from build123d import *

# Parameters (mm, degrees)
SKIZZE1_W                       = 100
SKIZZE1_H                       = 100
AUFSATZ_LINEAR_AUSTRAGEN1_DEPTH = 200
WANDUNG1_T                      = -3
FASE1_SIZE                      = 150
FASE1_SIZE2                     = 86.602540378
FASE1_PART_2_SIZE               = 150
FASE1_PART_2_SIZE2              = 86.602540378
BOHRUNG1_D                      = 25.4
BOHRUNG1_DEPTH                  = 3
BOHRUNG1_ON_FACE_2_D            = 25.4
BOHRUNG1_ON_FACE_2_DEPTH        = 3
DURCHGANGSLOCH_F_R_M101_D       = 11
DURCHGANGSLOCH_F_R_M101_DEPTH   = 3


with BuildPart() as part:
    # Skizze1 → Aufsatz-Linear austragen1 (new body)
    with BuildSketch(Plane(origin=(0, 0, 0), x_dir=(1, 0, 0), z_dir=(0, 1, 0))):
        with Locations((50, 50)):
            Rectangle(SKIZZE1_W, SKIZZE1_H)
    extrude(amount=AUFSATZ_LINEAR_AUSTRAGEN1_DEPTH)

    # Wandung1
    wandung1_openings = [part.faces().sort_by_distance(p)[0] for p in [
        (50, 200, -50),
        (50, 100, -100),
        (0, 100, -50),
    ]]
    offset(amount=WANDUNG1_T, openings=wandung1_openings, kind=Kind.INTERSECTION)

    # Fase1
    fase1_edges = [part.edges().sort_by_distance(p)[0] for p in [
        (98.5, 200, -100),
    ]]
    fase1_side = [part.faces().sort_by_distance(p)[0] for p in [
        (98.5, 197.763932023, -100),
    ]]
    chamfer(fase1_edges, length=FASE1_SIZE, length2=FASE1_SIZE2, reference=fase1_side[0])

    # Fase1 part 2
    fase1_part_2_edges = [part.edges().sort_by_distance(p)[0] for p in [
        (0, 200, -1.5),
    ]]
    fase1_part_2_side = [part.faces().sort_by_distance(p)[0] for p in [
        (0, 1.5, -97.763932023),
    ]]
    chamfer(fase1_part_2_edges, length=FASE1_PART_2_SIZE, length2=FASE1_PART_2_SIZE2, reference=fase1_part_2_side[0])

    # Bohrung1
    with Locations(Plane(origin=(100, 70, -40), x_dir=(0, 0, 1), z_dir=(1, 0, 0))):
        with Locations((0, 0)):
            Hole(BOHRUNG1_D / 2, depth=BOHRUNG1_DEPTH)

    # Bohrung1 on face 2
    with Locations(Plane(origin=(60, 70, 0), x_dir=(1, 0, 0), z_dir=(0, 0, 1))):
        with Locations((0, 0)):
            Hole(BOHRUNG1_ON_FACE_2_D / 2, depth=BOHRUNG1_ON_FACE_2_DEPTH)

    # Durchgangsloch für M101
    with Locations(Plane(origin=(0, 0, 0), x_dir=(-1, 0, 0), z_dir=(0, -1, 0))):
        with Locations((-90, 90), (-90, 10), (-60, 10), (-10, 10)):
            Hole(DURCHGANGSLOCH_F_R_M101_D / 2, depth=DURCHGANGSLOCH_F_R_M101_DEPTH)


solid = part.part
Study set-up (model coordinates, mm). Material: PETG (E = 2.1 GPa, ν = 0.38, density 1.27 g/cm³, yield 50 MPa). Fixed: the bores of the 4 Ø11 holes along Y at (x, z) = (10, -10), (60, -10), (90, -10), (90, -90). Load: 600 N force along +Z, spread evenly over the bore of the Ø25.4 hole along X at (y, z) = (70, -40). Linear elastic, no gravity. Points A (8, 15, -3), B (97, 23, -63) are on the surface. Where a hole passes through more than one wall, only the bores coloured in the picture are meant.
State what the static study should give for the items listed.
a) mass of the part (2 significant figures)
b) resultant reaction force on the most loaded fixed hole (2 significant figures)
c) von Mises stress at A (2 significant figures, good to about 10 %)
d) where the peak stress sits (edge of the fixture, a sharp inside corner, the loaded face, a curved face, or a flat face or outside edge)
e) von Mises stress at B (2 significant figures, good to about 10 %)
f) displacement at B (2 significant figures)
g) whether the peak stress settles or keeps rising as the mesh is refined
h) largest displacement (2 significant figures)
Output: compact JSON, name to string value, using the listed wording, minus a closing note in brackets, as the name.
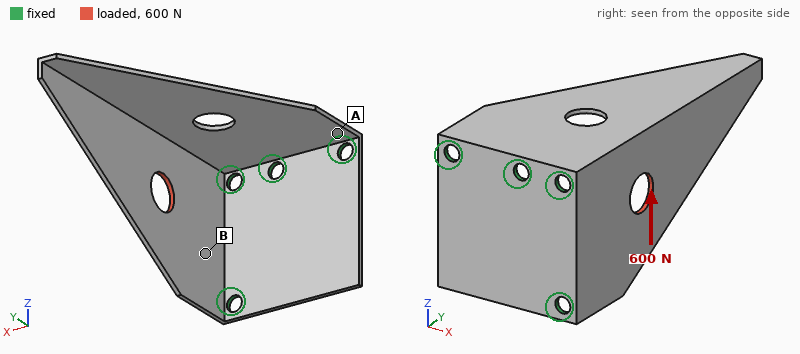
{"mass of the part": "130 g", "resultant reaction force on the most loaded fixed hole": "570 N", "von Mises stress at A": "2.1 MPa", "where the peak stress sits": "edge of the fixture", "von Mises stress at B": "5.2 MPa", "displacement at B": "0.27 mm", "whether the peak stress settles or keeps rising as the mesh is refined": "keeps rising", "largest displacement": "1.2 mm"}
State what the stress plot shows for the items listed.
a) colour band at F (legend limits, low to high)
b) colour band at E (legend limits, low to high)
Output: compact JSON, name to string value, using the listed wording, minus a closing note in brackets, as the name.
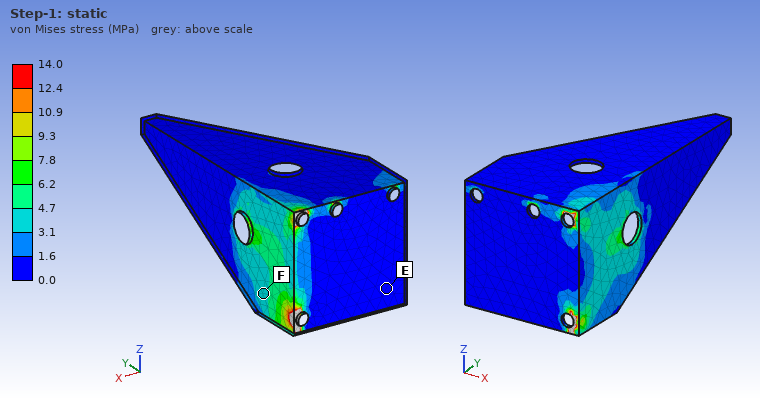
{"colour band at F": "3.1 to 4.7 MPa", "colour band at E": "0.0 to 1.6 MPa"}
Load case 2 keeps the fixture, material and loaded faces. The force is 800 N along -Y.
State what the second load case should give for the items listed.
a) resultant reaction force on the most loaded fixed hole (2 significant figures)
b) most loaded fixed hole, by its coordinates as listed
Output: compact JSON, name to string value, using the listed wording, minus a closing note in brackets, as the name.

{"resultant reaction force on the most loaded fixed hole": "470 N", "most loaded fixed hole, by its coordinates as listed": "(90, -10)"}
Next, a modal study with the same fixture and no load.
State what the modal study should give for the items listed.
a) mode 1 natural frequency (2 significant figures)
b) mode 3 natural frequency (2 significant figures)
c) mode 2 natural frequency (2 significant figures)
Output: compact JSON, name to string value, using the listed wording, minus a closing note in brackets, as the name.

{"mode 1 natural frequency": "90 Hz", "mode 3 natural frequency": "190 Hz", "mode 2 natural frequency": "170 Hz"}
